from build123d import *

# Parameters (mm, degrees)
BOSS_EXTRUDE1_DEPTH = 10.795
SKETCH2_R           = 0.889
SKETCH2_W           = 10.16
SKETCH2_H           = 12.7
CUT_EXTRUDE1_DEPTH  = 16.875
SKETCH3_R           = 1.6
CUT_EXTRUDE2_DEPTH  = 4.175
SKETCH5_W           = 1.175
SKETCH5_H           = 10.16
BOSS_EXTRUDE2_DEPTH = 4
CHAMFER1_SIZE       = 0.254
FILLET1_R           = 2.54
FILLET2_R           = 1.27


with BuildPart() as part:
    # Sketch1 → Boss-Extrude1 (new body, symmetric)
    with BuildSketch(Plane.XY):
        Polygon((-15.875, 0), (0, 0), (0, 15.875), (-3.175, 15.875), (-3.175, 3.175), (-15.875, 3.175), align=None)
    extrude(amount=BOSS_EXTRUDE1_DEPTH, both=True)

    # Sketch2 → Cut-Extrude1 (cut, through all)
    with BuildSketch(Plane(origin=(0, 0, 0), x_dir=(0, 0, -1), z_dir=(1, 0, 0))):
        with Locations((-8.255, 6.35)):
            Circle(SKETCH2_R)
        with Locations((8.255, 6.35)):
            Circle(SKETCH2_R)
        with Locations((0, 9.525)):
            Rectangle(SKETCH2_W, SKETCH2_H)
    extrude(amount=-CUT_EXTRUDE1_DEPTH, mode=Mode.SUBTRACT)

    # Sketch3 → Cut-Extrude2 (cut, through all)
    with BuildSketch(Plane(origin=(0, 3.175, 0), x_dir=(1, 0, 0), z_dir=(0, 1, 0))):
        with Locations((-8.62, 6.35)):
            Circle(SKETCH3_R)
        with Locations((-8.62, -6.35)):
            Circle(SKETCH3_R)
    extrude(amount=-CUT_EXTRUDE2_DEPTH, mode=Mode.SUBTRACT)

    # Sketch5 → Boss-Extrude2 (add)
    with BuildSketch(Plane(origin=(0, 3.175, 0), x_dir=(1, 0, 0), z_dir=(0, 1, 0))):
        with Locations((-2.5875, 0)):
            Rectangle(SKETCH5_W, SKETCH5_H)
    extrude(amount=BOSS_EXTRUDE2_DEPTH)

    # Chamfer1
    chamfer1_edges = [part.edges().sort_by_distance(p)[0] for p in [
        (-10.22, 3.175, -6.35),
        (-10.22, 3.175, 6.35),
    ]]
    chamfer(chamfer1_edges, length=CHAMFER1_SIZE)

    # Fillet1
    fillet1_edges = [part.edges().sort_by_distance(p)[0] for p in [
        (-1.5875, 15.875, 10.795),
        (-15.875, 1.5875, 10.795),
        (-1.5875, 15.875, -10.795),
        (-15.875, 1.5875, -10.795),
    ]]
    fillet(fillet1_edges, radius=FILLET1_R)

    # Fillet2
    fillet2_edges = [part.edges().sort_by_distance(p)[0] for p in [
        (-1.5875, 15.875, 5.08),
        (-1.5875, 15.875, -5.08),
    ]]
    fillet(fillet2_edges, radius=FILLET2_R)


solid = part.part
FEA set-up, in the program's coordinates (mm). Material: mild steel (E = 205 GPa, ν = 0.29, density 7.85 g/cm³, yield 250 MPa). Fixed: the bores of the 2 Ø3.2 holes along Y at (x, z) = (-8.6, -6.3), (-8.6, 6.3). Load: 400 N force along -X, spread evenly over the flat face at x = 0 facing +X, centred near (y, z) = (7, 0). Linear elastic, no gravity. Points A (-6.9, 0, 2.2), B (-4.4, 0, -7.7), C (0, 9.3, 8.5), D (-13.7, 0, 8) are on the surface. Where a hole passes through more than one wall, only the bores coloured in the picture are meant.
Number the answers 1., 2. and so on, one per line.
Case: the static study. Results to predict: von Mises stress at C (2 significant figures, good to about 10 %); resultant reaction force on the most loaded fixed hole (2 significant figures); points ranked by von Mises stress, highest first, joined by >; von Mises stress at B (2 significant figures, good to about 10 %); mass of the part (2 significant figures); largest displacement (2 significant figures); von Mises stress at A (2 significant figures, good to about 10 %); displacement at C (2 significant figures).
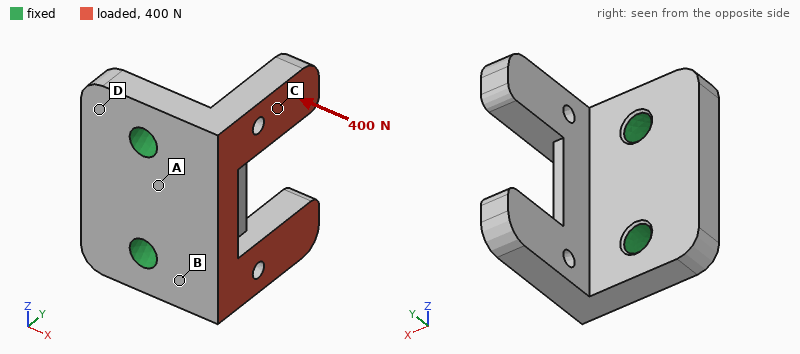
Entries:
1. 21 MPa
2. 200 N
3. B > A > C > D
4. 57 MPa
5. 12 g
6. 34 µm
7. 32 MPa
8. 17 µm
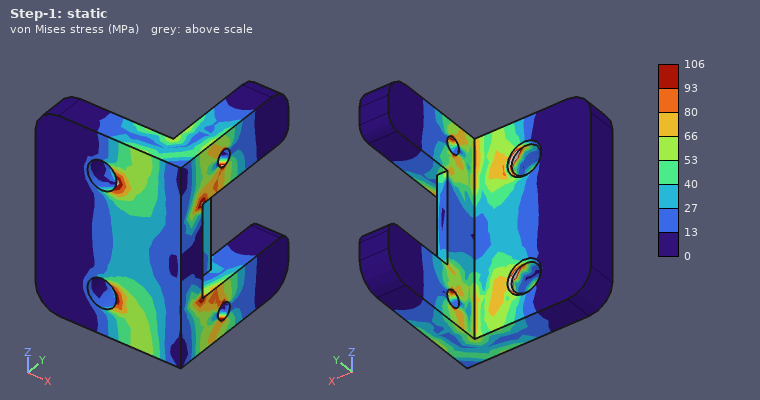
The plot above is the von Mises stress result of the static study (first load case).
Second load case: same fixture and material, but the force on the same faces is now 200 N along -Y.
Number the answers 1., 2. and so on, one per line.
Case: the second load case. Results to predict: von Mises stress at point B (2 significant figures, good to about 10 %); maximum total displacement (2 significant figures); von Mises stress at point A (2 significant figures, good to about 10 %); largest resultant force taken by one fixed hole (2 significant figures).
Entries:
1. 26 MPa
2. 11 µm
3. 20 MPa
4. 100 N
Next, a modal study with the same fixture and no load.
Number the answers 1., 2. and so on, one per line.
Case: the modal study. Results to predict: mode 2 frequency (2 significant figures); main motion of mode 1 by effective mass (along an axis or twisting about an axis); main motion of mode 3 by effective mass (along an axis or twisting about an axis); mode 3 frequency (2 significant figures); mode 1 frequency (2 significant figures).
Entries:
1. 10 kHz
2. along X
3. along Z
4. 18 kHz
5. 9200 Hz
